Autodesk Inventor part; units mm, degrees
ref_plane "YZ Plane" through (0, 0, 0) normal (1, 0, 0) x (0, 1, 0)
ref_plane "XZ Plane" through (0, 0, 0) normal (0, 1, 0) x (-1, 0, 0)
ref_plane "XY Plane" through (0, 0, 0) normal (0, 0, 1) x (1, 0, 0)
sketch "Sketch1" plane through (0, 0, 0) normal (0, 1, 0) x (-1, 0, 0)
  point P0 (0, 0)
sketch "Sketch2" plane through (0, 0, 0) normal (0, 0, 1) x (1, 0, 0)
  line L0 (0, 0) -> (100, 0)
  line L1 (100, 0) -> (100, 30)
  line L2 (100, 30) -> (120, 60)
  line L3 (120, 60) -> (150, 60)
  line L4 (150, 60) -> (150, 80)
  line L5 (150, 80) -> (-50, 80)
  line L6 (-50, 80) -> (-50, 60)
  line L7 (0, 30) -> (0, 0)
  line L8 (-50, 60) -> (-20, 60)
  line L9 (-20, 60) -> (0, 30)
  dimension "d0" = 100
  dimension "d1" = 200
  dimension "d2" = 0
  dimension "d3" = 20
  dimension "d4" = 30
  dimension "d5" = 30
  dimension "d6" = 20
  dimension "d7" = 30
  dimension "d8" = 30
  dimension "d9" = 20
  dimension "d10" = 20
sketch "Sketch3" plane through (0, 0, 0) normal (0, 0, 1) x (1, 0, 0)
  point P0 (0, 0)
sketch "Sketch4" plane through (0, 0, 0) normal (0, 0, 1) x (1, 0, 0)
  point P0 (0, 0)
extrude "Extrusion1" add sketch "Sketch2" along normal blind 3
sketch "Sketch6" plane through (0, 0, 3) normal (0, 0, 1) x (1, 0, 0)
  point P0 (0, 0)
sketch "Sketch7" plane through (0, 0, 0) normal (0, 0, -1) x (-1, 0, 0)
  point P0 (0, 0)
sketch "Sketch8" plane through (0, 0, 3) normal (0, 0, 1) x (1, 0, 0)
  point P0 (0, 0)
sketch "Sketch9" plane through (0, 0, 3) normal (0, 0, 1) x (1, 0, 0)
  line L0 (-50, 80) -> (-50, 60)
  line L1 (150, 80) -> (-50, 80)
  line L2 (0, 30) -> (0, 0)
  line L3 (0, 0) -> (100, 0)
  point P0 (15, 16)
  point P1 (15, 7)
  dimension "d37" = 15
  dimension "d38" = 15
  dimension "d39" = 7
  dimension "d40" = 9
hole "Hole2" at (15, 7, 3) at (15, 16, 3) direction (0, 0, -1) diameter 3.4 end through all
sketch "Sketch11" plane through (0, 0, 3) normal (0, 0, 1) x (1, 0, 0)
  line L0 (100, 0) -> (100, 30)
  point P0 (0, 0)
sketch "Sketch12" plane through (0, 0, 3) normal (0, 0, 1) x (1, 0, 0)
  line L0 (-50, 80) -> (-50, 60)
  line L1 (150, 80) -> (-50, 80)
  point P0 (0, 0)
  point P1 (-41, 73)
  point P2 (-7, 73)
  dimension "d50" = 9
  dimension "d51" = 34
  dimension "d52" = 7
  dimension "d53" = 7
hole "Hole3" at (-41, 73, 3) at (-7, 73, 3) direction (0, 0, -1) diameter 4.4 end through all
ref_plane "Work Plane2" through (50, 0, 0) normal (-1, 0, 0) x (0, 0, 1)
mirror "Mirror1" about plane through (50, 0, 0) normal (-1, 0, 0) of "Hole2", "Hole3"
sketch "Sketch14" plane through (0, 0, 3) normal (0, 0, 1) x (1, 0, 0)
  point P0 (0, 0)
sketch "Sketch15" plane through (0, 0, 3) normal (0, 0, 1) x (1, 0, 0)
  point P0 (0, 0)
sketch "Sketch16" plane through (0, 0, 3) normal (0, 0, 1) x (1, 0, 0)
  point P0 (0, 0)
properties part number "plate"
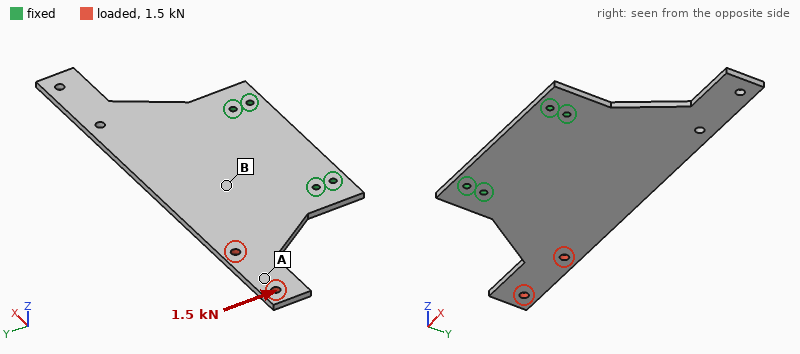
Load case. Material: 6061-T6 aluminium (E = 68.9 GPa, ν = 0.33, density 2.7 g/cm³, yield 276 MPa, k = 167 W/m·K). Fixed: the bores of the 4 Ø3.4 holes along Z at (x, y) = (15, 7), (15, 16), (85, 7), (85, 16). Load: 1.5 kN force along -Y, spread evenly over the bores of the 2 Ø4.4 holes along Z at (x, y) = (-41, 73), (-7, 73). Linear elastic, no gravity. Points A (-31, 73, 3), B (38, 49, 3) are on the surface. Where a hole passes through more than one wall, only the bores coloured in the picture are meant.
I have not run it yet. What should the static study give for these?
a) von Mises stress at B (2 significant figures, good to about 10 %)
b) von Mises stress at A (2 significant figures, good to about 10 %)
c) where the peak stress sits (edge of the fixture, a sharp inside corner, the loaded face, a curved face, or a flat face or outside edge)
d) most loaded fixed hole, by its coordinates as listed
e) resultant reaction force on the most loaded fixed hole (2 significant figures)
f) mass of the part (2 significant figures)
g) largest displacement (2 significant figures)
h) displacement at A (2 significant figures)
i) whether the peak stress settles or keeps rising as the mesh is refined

11 MPa
32 MPa
a sharp inside corner
(15, 16)
1.6 kN
85 g
0.20 mm
0.11 mm
keeps rising
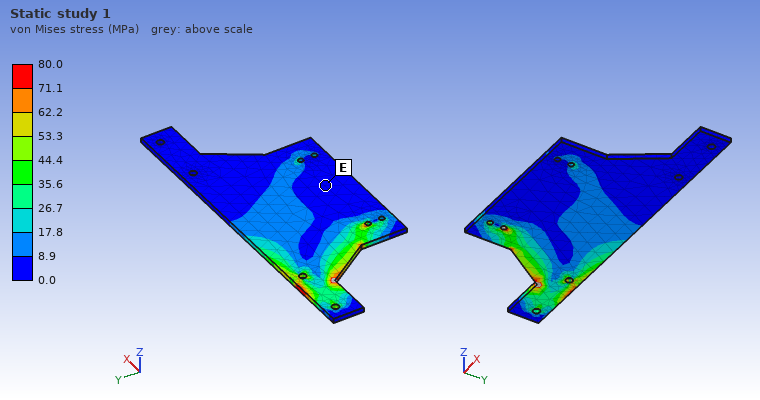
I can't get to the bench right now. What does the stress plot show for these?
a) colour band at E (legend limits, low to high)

0.0 to 8.9 MPa
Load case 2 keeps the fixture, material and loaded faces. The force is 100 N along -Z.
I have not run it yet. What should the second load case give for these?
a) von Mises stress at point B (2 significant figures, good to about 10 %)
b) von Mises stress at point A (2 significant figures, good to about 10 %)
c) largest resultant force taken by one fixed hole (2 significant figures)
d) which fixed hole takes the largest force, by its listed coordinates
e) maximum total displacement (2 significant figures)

34 MPa
20 MPa
380 N
(15, 16)
2.4 mm
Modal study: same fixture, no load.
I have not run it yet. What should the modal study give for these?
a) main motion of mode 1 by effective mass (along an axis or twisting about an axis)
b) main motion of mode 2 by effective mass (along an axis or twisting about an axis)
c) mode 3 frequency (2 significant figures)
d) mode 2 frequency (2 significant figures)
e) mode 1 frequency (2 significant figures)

along Z
twisting about Y
700 Hz
420 Hz
380 Hz
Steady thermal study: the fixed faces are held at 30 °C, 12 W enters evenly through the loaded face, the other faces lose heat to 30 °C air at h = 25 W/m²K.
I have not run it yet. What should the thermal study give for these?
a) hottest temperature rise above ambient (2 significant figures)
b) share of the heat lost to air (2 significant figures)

43 K
37 %
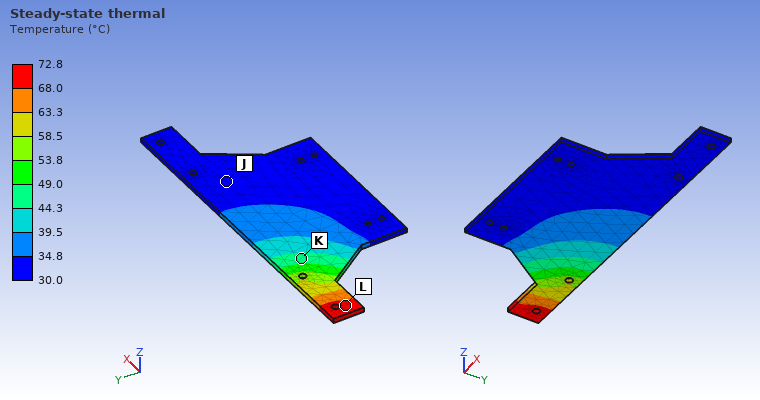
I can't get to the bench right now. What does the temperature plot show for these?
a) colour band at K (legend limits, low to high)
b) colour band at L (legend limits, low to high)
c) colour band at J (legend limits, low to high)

44.3 to 49.0 °C
68.0 to 72.8 °C
30.0 to 34.8 °C
